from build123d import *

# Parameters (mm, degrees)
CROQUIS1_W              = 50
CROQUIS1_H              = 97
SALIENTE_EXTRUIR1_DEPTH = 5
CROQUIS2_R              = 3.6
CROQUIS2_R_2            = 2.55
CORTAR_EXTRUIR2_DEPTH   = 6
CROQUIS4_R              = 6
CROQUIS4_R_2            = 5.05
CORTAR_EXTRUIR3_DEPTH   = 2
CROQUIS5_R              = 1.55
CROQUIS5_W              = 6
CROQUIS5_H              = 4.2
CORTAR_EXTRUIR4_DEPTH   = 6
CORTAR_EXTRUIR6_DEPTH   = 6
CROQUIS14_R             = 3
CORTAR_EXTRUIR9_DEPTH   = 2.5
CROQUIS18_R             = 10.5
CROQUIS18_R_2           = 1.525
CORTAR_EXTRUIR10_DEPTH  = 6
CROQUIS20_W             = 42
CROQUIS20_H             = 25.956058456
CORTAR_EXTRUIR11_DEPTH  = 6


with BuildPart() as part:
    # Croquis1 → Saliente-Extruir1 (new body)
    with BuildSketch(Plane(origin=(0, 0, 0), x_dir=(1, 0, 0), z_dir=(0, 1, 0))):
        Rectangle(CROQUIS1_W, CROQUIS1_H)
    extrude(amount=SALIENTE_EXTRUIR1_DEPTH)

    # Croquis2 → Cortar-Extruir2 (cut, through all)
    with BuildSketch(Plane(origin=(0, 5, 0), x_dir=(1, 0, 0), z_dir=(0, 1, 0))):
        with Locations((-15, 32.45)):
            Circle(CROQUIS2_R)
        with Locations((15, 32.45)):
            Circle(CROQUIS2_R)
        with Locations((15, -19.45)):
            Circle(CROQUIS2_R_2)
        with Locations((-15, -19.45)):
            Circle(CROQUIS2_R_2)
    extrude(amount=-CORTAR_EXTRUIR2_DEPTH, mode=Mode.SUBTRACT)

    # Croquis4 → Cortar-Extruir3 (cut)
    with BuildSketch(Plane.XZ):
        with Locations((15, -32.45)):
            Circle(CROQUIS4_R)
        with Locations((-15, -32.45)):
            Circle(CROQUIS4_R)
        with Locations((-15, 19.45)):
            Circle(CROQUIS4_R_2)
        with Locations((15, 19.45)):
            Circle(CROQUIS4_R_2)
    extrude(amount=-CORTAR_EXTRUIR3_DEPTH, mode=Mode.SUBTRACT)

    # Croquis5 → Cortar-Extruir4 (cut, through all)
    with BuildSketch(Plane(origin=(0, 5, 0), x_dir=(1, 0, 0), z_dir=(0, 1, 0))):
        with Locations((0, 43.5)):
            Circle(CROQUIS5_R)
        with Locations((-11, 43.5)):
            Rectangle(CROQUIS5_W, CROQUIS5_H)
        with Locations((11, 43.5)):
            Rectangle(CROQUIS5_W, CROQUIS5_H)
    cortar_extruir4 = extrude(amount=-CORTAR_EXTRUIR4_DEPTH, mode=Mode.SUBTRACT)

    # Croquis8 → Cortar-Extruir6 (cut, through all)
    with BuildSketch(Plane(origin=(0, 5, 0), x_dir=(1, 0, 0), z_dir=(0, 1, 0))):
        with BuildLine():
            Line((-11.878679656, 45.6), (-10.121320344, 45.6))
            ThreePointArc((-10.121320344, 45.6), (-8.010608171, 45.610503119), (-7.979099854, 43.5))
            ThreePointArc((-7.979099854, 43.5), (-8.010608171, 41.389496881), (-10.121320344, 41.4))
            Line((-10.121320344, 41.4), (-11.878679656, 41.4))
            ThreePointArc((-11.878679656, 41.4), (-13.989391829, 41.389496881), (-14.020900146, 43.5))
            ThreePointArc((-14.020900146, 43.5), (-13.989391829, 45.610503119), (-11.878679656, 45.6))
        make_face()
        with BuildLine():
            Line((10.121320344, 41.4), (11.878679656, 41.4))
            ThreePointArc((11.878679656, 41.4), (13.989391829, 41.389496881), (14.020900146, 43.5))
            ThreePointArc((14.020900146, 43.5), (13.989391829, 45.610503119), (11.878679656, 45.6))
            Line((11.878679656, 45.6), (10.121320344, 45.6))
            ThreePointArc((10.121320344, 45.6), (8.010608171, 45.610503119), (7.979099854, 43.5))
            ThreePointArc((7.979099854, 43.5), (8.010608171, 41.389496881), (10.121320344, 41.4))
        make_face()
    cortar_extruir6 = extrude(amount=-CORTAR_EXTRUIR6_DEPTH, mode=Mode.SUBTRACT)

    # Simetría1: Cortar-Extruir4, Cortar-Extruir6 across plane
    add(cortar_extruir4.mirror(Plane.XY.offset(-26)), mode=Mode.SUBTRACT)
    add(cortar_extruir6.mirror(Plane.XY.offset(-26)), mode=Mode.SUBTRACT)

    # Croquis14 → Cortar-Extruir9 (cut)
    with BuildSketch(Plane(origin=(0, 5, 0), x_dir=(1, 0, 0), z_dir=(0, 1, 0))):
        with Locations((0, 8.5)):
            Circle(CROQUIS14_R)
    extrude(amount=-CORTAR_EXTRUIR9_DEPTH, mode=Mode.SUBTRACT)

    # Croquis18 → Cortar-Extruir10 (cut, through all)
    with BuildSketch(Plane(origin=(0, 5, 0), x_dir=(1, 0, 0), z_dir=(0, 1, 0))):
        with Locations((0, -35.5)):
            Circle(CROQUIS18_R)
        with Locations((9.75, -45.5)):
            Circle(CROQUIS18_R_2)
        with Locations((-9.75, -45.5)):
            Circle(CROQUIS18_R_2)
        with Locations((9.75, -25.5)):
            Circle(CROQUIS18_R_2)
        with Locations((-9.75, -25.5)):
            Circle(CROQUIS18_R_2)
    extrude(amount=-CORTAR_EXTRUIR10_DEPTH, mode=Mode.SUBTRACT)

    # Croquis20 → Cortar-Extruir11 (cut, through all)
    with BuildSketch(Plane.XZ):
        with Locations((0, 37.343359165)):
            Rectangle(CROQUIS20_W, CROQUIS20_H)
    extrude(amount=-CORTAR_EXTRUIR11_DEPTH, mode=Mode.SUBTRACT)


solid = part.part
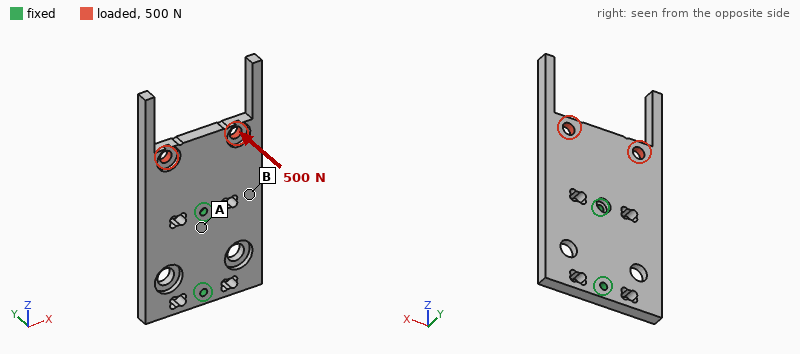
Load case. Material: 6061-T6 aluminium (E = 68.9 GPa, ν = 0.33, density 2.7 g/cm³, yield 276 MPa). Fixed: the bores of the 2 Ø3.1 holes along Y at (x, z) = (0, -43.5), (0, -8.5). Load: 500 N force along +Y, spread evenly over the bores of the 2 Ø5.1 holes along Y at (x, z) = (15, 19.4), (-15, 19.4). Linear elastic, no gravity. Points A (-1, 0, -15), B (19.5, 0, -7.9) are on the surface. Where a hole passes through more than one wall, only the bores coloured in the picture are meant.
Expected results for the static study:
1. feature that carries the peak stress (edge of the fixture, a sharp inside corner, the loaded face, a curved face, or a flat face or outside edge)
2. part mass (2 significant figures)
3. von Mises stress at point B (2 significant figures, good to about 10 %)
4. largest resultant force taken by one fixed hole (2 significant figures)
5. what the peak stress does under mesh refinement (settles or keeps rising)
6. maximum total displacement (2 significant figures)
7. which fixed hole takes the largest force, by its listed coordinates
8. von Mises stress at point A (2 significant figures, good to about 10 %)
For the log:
edge of the fixture
47 g
56 MPa
1.0 kN
keeps rising
0.50 mm
(0, -8.5)
24 MPa
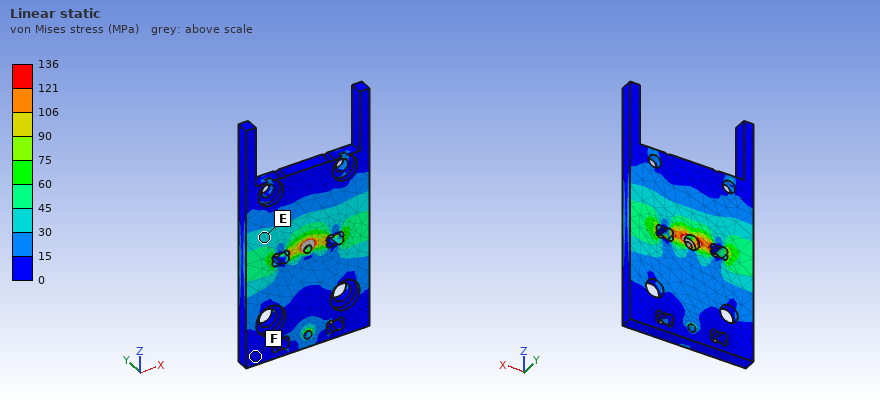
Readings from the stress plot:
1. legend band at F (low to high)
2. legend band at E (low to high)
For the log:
0 to 15 MPa
30 to 45 MPa
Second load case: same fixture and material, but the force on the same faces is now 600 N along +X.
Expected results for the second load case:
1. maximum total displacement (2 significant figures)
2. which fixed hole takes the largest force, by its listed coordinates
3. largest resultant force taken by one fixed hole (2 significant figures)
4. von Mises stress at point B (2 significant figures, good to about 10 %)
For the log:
55 µm
(0, -8.5)
1.0 kN
6.0 MPa
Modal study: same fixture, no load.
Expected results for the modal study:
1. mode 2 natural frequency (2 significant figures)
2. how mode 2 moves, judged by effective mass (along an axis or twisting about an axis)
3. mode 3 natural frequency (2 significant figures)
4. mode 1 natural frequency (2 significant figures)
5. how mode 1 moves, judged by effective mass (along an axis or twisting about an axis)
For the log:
1900 Hz
twisting about Z
3600 Hz
1800 Hz
along Y
